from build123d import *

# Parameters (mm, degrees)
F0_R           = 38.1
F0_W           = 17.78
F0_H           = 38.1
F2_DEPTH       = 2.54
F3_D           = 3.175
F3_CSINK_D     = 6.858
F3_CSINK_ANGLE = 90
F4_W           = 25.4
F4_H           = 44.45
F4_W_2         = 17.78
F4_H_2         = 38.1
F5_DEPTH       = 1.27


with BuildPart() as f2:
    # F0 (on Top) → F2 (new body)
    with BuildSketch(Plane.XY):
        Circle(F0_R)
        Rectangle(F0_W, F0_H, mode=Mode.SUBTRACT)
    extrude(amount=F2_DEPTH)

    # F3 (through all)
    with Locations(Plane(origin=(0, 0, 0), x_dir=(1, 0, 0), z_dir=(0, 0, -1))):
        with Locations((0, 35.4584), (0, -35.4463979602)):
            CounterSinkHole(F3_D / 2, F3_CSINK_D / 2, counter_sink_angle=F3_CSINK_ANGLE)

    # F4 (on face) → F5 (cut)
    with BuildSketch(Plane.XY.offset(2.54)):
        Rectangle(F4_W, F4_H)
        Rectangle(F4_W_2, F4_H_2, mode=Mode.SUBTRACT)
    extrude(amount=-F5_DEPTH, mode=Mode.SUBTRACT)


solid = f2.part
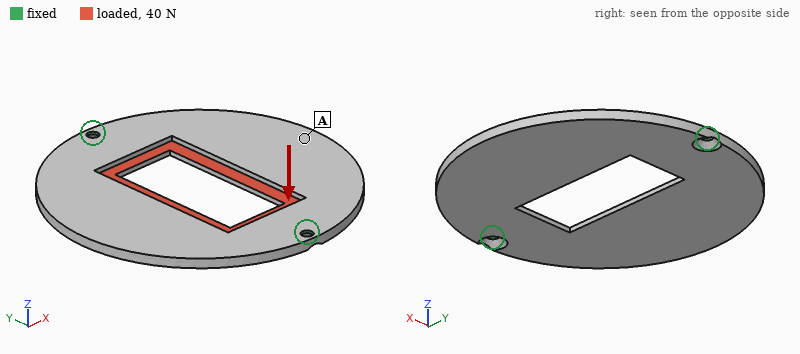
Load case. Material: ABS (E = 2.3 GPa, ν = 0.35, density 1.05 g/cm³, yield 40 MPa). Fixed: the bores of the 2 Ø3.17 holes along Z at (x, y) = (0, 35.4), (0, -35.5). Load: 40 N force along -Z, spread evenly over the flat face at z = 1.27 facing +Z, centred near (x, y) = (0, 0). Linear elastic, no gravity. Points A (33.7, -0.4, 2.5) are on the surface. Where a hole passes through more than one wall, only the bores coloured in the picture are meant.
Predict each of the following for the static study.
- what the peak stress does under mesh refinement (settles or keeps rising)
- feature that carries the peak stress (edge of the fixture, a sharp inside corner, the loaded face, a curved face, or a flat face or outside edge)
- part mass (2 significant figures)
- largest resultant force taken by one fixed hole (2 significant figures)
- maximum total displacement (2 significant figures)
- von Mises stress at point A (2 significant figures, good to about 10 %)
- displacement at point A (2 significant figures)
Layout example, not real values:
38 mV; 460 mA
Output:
keeps rising; edge of the fixture; 9.7 g; 49 N; 1.0 mm; 3.4 MPa; 0.78 mm
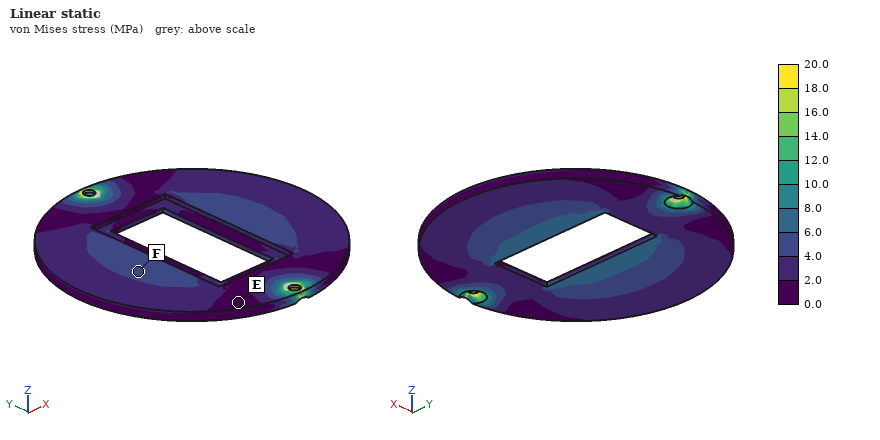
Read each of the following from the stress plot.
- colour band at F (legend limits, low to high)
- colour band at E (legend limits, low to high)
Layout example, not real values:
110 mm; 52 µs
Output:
4.0 to 6.0 MPa; 0.0 to 2.0 MPa
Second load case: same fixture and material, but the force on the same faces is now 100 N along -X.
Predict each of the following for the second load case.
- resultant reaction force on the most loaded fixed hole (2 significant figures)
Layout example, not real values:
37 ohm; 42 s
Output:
50 N
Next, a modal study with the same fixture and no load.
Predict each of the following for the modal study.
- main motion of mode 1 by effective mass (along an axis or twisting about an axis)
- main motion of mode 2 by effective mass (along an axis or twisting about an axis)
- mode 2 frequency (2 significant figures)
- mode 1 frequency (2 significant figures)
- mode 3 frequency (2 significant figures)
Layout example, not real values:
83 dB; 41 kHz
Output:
twisting about Y; along Z; 310 Hz; 190 Hz; 700 Hz
